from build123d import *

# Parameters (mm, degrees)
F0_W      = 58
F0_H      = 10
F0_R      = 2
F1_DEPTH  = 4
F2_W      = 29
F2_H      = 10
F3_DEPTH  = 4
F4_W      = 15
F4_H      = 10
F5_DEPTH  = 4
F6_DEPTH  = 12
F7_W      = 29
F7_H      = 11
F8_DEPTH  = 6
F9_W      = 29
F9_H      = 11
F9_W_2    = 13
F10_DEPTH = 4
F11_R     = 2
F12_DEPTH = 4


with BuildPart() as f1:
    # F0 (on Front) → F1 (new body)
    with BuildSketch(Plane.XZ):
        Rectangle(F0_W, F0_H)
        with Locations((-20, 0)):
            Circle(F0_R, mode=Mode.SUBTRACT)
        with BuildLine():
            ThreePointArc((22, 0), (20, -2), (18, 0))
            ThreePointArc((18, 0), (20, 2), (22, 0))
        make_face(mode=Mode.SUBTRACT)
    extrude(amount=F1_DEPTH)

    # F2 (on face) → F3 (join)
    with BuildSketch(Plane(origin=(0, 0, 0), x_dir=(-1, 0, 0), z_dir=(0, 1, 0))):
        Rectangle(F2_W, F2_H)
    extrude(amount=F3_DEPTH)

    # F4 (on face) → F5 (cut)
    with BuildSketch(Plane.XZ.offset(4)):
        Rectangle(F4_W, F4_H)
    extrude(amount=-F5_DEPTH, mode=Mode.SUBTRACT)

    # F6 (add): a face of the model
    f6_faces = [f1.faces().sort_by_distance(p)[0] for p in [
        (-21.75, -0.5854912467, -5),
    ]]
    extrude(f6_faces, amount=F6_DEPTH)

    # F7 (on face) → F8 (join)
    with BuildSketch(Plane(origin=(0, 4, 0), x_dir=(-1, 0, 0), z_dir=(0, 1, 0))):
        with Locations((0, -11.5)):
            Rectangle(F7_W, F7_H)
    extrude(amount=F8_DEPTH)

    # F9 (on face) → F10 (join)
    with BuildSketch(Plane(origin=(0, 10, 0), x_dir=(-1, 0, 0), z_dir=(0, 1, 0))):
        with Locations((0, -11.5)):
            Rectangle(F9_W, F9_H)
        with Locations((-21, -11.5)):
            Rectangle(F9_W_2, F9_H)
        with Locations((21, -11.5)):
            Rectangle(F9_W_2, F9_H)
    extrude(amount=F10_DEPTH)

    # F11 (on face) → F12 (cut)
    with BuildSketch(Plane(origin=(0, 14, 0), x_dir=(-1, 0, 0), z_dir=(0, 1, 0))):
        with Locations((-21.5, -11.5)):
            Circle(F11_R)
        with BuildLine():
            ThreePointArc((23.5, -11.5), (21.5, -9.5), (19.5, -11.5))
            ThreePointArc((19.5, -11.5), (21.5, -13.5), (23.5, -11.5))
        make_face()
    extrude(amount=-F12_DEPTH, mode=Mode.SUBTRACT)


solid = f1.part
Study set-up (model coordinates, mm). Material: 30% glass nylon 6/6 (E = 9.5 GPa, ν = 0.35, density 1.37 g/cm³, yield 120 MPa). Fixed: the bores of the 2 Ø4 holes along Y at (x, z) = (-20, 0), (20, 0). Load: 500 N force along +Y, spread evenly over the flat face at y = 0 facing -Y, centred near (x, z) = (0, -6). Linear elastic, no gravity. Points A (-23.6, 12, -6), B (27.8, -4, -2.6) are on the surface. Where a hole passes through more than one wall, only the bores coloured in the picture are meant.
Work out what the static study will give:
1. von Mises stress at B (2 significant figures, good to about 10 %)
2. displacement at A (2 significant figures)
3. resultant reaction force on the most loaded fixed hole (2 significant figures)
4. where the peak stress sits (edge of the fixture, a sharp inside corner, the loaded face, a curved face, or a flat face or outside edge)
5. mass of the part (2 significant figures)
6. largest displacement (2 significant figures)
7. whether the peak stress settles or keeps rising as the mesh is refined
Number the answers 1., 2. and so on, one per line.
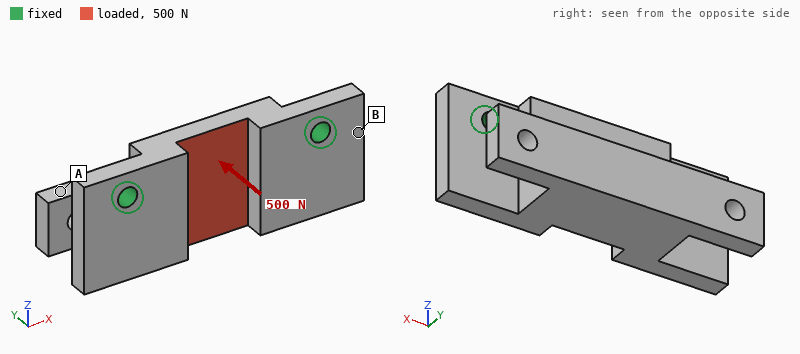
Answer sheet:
1. 9.3 MPa
2. 0.10 mm
3. 330 N
4. edge of the fixture
5. 14 g
6. 0.17 mm
7. keeps rising
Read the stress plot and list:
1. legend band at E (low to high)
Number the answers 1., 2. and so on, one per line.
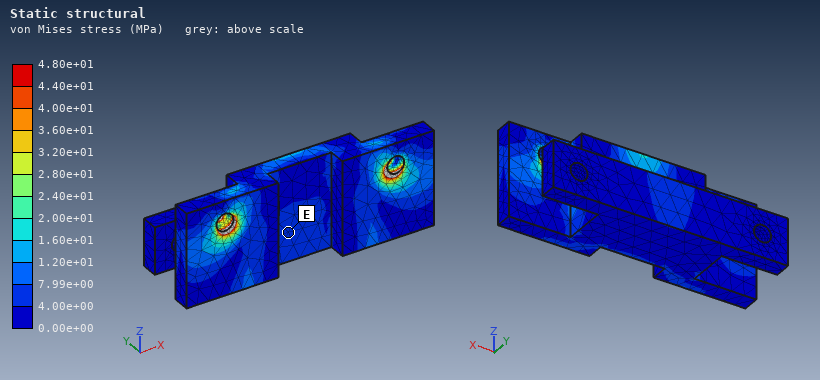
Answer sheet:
1. 4.00e+00 to 7.99e+00 MPa
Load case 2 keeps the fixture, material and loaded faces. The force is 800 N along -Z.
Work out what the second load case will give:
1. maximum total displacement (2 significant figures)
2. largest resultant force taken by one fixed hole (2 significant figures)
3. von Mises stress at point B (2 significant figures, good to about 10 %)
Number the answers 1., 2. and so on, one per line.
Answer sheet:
1. 0.12 mm
2. 420 N
3. 5.0 MPa
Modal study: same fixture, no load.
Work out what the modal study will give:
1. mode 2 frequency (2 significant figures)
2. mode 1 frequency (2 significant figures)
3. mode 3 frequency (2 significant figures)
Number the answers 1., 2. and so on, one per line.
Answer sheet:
1. 4800 Hz
2. 2100 Hz
3. 6400 Hz
